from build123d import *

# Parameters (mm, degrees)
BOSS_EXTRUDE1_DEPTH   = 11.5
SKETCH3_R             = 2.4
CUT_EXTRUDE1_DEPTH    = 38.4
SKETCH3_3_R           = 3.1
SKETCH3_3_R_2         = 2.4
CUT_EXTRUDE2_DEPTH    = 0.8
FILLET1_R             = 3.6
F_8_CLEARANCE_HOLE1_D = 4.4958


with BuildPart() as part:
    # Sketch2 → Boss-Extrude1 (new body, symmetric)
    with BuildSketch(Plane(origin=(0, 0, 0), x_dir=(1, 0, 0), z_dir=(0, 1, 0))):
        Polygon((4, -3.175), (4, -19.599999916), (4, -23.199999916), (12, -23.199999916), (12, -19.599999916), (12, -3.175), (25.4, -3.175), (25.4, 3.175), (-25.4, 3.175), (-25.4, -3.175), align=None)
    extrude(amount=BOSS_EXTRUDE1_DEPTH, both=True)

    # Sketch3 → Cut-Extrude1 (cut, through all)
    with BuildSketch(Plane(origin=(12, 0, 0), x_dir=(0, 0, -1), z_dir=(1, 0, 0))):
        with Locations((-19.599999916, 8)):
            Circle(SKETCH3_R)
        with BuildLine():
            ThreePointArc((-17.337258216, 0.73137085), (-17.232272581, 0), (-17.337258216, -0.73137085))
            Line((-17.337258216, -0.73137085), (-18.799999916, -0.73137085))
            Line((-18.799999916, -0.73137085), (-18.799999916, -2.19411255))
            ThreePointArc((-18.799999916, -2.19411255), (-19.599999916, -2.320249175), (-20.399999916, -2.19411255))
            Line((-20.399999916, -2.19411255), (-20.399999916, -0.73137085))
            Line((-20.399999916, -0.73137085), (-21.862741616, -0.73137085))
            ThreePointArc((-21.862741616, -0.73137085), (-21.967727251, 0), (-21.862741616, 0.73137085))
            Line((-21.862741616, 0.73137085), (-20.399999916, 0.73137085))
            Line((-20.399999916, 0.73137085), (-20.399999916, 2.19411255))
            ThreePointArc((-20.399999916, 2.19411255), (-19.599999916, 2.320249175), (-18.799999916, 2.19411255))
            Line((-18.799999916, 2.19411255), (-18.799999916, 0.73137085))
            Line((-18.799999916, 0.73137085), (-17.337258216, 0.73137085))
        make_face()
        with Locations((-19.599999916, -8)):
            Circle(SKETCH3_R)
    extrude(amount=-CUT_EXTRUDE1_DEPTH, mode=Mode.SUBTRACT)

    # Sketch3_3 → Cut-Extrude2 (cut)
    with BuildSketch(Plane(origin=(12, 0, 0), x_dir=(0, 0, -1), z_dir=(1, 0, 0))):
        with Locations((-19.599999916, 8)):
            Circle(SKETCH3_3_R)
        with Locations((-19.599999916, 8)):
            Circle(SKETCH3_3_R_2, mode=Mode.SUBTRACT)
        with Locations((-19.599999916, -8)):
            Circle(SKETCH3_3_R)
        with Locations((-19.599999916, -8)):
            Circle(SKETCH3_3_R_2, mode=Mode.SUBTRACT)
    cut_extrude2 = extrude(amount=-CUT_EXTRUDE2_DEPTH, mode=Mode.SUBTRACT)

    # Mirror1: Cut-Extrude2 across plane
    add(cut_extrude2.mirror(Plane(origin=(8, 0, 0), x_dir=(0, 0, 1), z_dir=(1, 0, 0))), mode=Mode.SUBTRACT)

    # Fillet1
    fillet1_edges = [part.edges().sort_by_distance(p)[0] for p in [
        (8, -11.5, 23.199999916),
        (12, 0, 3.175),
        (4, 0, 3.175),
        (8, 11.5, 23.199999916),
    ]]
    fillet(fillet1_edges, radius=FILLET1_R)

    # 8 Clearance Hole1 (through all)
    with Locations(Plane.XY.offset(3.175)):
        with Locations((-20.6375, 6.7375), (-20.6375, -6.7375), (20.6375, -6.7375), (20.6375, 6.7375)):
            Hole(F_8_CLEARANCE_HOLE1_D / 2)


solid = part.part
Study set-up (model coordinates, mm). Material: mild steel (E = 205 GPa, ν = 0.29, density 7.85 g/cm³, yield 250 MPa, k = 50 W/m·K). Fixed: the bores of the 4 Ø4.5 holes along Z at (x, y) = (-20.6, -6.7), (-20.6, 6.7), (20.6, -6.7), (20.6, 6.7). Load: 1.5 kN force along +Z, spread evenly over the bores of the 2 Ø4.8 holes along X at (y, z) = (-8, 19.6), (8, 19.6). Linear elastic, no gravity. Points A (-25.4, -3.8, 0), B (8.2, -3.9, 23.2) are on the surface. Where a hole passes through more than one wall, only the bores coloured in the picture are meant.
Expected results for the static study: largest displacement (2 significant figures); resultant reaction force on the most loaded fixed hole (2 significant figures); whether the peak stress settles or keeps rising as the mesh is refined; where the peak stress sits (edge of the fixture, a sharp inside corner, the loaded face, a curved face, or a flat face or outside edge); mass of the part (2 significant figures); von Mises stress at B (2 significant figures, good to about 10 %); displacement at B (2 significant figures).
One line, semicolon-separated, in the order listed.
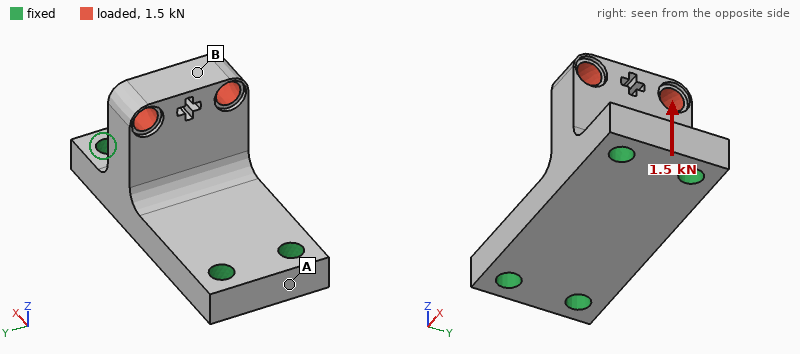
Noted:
6.6 µm; 570 N; keeps rising; edge of the fixture; 81 g; 18 MPa; 5.3 µm
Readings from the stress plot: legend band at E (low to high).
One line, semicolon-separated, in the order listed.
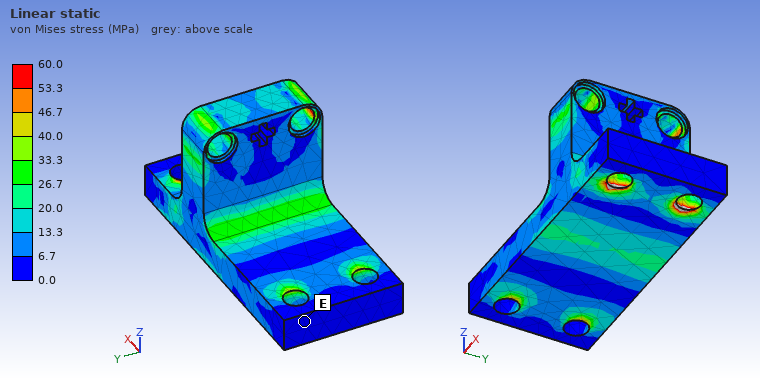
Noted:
0.0 to 6.7 MPa
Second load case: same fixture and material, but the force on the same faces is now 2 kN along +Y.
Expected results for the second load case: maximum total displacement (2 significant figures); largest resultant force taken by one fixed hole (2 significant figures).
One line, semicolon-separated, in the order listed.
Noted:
29 µm; 2.2 kN
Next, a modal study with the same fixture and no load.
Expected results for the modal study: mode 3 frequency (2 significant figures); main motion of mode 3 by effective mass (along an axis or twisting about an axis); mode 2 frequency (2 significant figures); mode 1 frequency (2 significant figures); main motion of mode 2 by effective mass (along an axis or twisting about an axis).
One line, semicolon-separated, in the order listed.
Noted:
20 kHz; along Z; 12 kHz; 11 kHz; along Y
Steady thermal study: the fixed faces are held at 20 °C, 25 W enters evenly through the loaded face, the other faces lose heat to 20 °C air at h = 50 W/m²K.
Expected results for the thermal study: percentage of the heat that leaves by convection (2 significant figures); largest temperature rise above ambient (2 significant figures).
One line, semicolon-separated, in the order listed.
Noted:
18 %; 79 K
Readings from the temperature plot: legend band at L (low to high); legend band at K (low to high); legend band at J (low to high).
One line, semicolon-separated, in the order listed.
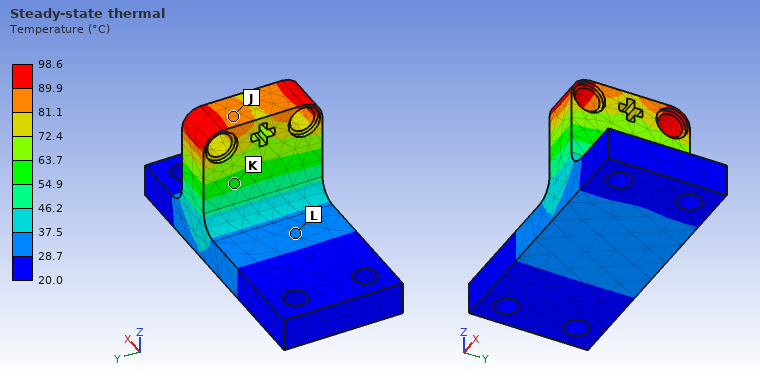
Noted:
28.7 to 37.5 °C; 54.9 to 63.7 °C; 81.1 to 89.9 °C
